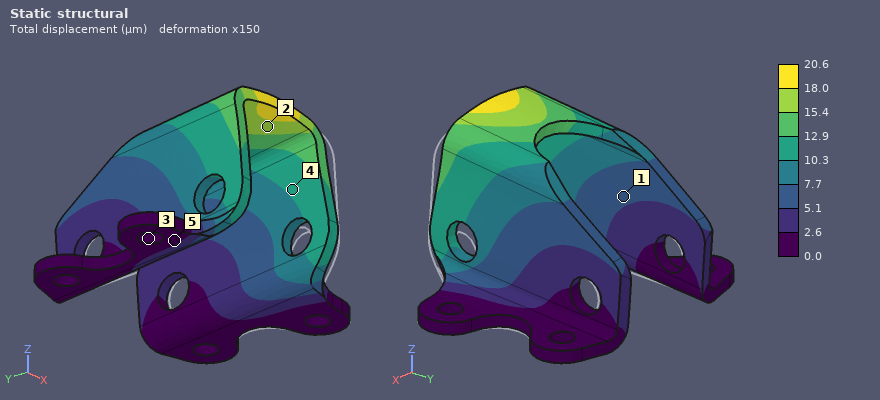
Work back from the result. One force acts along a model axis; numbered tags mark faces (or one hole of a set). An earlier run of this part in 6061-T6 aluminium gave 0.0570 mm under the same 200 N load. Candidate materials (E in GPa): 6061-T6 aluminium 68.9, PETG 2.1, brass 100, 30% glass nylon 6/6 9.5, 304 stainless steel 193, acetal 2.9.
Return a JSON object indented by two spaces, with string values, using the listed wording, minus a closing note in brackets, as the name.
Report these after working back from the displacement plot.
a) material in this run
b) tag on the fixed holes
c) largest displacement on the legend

{
  "material in this run": "304 stainless steel",
  "tag on the fixed holes": "3",
  "largest displacement on the legend": "20.6 µm"
}
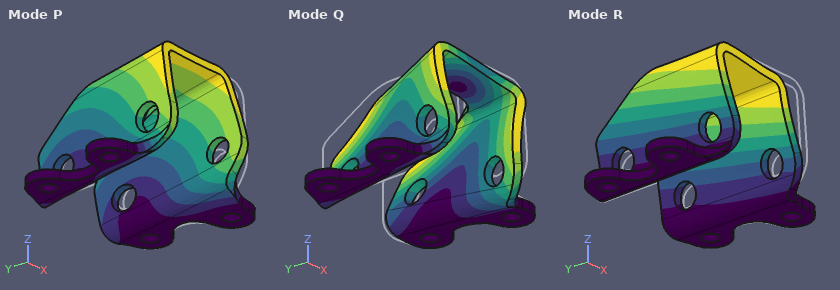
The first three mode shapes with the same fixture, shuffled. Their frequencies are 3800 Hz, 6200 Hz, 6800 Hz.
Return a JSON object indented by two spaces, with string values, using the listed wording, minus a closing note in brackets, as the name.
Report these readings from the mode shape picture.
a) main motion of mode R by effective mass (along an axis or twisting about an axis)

{
  "main motion of mode R by effective mass": "along X"
}
